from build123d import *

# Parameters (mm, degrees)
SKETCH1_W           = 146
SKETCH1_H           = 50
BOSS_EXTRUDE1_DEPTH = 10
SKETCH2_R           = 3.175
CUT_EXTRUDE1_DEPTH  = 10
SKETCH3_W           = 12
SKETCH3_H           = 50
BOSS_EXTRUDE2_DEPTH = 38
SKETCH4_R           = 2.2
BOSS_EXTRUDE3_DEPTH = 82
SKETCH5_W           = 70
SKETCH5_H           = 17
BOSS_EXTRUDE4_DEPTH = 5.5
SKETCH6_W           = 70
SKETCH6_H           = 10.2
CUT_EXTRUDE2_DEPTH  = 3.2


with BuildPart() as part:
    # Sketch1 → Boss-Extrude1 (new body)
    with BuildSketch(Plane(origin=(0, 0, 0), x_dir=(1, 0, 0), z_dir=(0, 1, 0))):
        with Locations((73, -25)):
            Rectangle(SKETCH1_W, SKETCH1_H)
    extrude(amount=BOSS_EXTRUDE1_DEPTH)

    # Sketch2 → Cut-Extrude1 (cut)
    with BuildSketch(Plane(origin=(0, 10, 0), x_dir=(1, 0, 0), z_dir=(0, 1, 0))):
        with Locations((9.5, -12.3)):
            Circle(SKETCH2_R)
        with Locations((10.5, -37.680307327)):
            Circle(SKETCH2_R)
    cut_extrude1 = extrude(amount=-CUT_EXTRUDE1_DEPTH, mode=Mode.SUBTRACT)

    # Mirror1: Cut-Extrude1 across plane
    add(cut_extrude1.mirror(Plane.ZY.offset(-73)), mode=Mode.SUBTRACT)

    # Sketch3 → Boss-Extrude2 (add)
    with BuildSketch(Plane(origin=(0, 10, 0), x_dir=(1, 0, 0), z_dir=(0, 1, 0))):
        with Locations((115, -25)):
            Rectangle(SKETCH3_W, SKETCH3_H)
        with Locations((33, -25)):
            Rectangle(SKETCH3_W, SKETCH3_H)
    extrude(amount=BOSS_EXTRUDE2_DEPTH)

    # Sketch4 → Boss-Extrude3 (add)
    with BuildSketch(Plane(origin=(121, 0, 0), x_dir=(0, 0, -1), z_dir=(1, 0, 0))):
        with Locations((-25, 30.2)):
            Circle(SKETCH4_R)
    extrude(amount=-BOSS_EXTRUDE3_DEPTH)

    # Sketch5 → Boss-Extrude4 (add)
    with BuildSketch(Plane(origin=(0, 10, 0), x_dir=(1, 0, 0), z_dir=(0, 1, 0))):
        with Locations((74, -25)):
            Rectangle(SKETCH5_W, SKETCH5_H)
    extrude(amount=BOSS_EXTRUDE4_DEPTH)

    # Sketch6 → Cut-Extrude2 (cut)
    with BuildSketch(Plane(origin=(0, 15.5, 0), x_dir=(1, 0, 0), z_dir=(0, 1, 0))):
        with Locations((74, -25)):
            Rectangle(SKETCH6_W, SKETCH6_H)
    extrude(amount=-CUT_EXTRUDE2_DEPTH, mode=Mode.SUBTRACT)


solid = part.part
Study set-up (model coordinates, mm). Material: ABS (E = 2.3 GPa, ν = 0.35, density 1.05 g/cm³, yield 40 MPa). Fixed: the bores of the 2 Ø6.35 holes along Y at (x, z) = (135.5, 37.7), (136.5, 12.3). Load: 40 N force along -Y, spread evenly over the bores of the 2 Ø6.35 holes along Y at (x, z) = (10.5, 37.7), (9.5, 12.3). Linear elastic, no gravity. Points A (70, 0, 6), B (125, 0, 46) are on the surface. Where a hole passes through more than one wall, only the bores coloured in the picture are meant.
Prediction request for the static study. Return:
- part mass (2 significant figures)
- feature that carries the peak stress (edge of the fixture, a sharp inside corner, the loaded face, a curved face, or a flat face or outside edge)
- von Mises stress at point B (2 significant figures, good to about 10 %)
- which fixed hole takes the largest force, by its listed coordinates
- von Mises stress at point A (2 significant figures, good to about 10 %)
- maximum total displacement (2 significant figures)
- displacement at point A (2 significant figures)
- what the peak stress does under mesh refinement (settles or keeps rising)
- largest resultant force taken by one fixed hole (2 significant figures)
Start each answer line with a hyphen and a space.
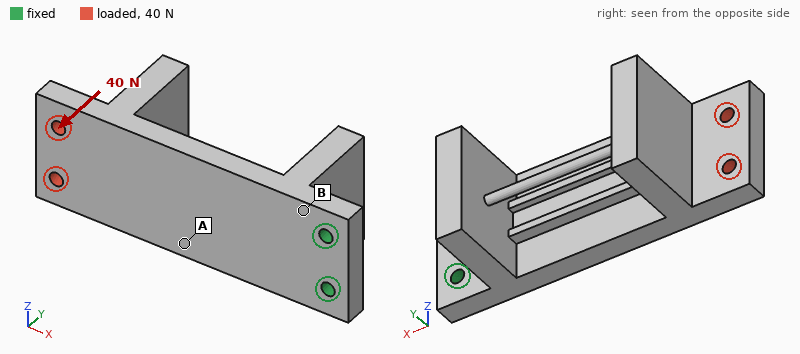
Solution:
- 130 g
- edge of the fixture
- 5.0 MPa
- (135.5, 37.7)
- 0.99 MPa
- 1.7 mm
- 0.65 mm
- keeps rising
- 26 N
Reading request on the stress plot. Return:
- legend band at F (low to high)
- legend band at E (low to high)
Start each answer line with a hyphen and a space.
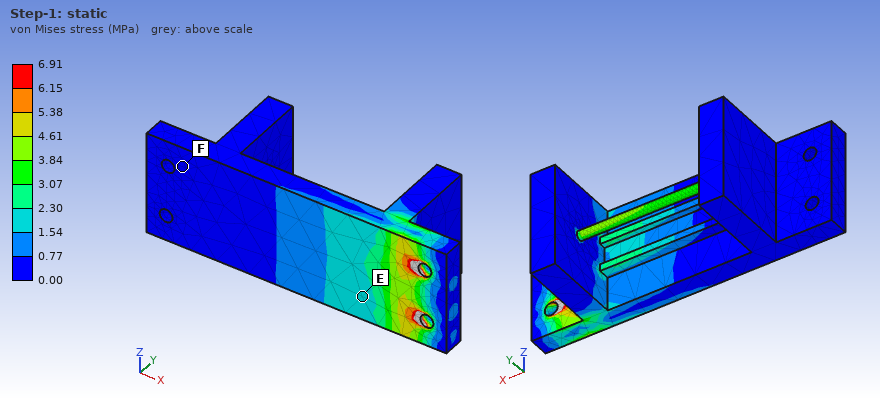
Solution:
- 0.00 to 0.77 MPa
- 1.54 to 2.30 MPa
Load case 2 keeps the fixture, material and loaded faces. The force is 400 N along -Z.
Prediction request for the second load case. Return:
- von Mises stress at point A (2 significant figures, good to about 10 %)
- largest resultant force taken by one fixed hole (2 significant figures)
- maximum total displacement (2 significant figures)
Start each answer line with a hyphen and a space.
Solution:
- 4.3 MPa
- 1.7 kN
- 1.6 mm
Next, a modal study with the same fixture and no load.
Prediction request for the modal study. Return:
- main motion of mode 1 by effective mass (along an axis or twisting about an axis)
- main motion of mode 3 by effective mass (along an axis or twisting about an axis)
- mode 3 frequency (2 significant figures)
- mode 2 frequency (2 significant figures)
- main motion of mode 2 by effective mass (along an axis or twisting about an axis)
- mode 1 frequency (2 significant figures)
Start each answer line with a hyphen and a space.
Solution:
- along Y
- along Z
- 540 Hz
- 370 Hz
- along Z
- 130 Hz
